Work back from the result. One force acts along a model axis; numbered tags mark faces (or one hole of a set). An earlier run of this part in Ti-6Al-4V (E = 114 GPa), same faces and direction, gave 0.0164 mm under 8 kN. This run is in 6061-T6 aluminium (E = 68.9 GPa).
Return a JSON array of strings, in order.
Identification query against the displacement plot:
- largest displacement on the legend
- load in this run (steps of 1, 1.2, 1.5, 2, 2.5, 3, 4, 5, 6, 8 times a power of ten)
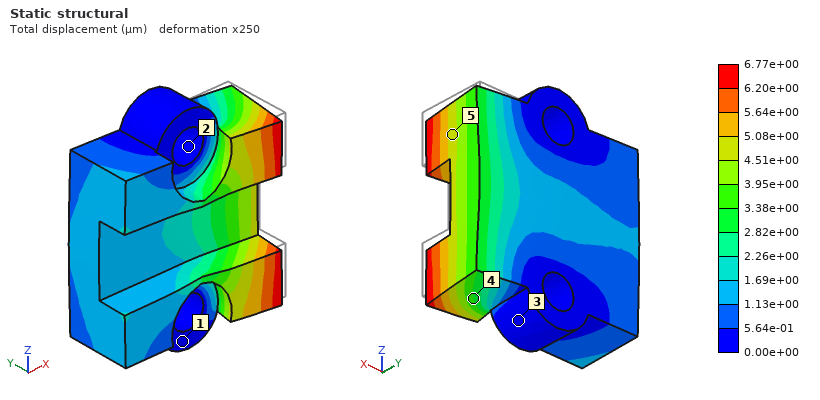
["6.77e+00 µm", "2 kN"]
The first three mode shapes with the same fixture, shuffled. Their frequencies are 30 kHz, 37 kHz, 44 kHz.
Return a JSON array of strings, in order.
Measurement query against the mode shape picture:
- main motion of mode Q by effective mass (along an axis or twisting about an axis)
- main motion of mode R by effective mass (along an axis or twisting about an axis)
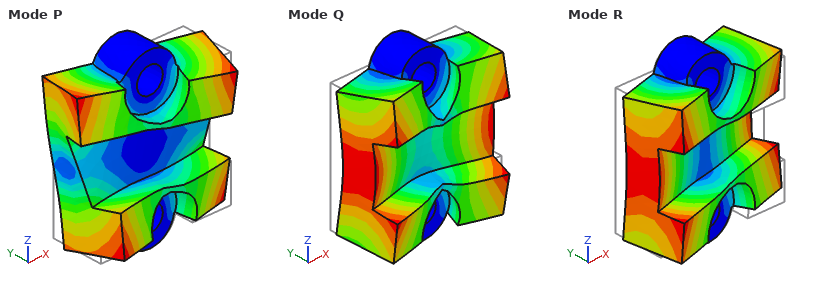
["along Y", "twisting about Z"]
